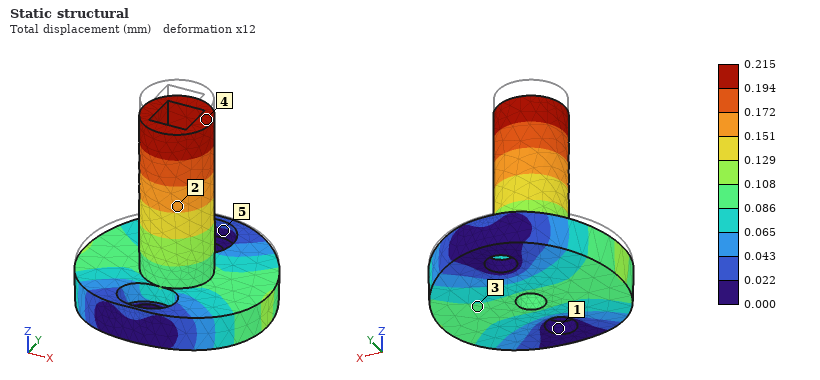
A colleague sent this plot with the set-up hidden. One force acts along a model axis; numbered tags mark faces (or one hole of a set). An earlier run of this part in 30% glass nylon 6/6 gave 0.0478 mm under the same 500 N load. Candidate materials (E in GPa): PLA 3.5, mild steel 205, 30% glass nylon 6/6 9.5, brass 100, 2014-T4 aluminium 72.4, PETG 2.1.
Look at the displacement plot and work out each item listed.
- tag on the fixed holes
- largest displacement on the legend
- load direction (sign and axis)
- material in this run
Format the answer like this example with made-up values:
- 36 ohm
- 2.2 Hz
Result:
- 1
- 0.215 mm
- -Z
- PETG
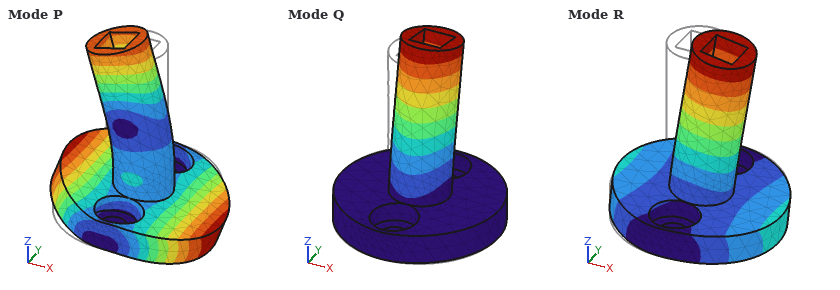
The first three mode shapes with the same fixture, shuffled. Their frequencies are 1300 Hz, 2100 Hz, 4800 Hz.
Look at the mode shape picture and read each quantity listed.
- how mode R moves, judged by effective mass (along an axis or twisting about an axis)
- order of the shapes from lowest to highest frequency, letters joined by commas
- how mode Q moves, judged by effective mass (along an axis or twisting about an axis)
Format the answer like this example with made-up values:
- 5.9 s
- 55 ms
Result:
- along X
- R, Q, P
- along Y
